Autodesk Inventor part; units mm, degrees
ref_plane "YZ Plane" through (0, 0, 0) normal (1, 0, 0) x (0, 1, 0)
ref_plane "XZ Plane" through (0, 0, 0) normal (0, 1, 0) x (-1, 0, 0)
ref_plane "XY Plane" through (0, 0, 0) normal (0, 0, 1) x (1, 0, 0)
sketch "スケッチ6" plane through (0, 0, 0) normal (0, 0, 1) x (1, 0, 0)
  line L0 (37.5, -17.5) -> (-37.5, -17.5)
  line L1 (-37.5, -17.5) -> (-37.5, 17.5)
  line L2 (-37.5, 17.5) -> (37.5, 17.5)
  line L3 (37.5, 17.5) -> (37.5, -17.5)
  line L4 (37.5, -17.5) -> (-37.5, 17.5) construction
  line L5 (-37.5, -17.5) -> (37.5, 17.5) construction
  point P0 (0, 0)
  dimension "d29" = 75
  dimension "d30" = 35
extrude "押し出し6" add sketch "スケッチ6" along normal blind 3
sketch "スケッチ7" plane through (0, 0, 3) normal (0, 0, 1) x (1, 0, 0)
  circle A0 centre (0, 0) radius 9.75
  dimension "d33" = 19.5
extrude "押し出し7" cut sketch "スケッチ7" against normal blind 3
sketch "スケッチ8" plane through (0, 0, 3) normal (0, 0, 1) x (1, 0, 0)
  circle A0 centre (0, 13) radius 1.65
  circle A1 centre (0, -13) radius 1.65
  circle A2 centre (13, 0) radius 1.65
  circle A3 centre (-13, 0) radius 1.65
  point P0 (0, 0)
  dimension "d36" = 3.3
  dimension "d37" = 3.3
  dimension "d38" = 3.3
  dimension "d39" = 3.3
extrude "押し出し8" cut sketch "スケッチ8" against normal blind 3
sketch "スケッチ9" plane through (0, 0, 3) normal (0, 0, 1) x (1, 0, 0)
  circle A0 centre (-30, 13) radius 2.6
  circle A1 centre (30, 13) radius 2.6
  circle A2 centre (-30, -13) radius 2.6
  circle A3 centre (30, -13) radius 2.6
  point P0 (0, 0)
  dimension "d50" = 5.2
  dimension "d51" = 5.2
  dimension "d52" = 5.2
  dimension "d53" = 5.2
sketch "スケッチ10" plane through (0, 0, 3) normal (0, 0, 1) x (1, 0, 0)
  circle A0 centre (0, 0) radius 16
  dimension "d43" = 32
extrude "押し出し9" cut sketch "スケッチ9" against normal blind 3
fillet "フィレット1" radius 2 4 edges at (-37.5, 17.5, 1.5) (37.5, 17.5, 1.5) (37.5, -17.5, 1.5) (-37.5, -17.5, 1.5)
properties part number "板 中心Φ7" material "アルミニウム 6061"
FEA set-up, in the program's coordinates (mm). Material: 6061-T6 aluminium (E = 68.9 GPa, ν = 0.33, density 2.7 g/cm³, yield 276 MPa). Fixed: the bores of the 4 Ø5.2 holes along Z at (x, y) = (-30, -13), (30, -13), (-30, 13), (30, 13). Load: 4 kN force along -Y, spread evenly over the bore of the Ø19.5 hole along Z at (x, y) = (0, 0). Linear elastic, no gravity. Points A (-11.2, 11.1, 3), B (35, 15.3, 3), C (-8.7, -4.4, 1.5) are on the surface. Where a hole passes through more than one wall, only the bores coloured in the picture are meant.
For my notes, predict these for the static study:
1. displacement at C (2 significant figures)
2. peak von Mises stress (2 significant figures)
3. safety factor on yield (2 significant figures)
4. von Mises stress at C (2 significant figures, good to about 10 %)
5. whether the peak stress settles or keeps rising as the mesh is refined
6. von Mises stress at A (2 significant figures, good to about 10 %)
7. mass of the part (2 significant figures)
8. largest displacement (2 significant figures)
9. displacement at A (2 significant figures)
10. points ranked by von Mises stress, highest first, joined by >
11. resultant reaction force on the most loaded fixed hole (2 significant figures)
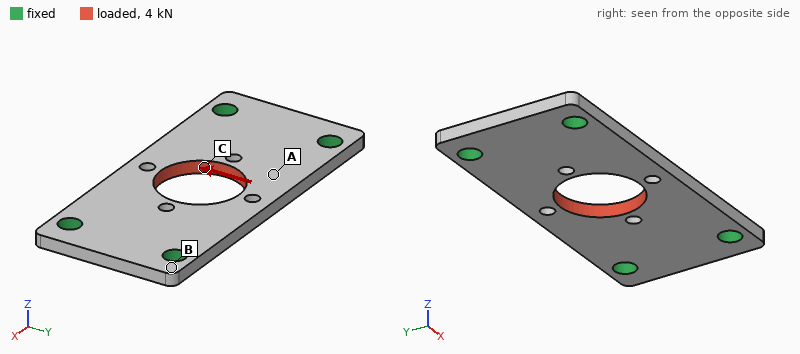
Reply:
24 µm
150 MPa
1.9
54 MPa
settles
32 MPa
18 g
35 µm
21 µm
C > A > B
1.4 kN
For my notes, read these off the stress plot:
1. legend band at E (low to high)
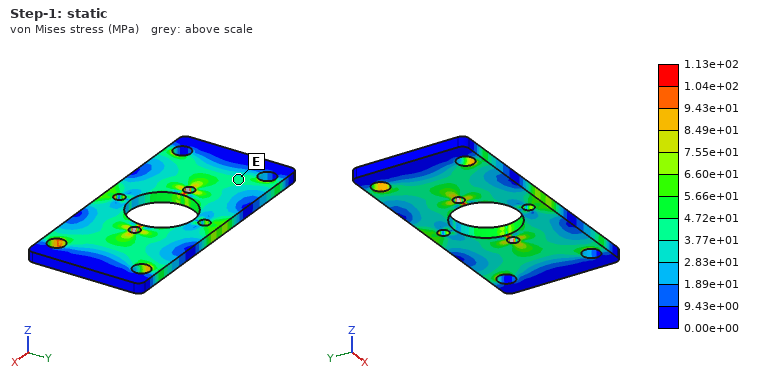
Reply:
3.77e+01 to 4.72e+01 MPa
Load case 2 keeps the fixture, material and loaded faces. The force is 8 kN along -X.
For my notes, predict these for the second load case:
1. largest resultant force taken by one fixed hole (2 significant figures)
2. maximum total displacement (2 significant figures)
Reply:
2.0 kN
19 µm
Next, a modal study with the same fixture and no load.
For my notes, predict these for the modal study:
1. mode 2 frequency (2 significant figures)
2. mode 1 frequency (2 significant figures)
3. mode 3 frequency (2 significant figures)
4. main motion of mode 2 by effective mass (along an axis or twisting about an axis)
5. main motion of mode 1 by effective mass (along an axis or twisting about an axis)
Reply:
6700 Hz
4900 Hz
11 kHz
twisting about X
along Z
